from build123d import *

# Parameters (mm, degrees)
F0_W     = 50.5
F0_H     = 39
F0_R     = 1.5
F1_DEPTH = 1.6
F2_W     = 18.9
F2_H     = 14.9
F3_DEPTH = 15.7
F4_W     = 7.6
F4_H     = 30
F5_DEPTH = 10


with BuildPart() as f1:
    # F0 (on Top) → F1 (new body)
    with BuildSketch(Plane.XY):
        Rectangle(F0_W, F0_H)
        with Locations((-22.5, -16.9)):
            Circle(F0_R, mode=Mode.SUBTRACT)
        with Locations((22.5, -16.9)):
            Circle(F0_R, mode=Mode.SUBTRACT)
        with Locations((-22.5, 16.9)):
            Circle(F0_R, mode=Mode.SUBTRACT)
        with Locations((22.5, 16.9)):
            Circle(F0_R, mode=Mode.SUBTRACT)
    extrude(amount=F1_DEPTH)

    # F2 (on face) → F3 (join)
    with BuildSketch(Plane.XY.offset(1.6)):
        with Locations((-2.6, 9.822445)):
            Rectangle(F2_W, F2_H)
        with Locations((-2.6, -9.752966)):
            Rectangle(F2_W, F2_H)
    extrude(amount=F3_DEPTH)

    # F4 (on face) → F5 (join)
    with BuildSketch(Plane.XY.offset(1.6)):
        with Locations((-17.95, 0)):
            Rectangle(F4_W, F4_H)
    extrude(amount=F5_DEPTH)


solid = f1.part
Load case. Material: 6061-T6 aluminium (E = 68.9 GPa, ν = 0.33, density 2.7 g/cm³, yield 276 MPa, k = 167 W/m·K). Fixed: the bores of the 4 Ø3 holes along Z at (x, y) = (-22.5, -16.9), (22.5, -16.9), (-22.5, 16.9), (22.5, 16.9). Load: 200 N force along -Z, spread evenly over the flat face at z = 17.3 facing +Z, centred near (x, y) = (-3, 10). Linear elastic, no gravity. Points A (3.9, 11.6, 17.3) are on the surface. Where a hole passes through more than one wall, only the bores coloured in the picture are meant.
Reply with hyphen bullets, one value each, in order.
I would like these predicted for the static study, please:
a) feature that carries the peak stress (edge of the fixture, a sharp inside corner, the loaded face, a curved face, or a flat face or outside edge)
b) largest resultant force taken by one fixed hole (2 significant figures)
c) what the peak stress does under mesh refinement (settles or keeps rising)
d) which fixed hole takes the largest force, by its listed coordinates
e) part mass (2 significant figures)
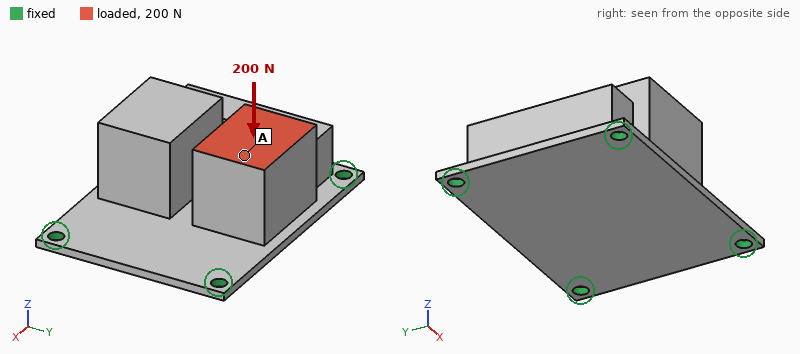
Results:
- edge of the fixture
- 120 N
- keeps rising
- (-22.5, 16.9)
- 38 g
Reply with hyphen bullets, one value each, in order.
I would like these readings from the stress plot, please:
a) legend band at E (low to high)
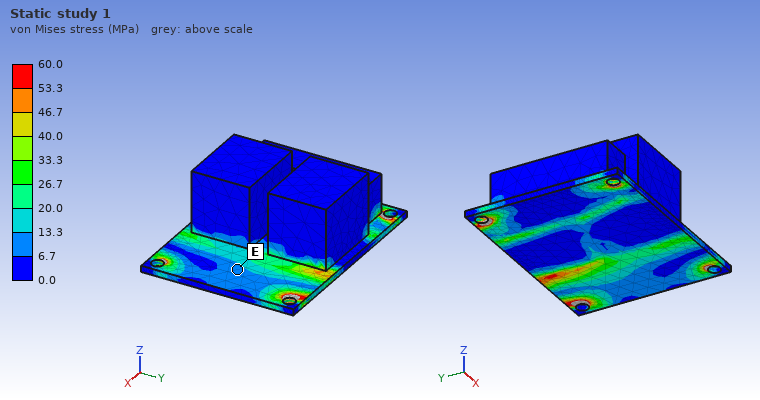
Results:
- 6.7 to 13.3 MPa
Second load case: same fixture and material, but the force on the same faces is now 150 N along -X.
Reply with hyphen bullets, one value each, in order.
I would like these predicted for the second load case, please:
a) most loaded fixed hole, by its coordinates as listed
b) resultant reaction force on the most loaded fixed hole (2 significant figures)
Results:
- (-22.5, 16.9)
- 71 N
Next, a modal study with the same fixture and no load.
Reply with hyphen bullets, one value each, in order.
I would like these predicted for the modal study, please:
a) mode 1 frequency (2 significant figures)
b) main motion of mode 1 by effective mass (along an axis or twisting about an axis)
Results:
- 2100 Hz
- along Z
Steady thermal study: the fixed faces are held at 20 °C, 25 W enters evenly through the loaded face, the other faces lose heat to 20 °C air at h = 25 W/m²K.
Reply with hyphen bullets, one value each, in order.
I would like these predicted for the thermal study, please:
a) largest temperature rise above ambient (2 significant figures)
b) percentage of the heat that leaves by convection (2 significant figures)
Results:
- 34 K
- 11 %
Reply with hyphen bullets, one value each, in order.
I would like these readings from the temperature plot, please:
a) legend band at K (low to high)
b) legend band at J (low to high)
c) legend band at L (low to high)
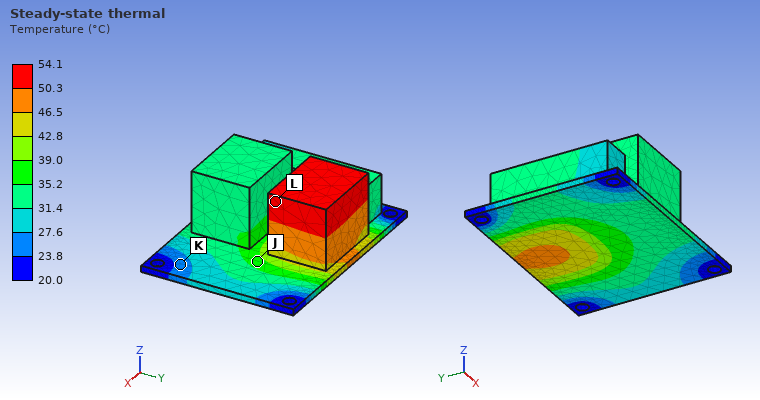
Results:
- 23.8 to 27.6 °C
- 35.2 to 39.0 °C
- 50.3 to 54.1 °C
